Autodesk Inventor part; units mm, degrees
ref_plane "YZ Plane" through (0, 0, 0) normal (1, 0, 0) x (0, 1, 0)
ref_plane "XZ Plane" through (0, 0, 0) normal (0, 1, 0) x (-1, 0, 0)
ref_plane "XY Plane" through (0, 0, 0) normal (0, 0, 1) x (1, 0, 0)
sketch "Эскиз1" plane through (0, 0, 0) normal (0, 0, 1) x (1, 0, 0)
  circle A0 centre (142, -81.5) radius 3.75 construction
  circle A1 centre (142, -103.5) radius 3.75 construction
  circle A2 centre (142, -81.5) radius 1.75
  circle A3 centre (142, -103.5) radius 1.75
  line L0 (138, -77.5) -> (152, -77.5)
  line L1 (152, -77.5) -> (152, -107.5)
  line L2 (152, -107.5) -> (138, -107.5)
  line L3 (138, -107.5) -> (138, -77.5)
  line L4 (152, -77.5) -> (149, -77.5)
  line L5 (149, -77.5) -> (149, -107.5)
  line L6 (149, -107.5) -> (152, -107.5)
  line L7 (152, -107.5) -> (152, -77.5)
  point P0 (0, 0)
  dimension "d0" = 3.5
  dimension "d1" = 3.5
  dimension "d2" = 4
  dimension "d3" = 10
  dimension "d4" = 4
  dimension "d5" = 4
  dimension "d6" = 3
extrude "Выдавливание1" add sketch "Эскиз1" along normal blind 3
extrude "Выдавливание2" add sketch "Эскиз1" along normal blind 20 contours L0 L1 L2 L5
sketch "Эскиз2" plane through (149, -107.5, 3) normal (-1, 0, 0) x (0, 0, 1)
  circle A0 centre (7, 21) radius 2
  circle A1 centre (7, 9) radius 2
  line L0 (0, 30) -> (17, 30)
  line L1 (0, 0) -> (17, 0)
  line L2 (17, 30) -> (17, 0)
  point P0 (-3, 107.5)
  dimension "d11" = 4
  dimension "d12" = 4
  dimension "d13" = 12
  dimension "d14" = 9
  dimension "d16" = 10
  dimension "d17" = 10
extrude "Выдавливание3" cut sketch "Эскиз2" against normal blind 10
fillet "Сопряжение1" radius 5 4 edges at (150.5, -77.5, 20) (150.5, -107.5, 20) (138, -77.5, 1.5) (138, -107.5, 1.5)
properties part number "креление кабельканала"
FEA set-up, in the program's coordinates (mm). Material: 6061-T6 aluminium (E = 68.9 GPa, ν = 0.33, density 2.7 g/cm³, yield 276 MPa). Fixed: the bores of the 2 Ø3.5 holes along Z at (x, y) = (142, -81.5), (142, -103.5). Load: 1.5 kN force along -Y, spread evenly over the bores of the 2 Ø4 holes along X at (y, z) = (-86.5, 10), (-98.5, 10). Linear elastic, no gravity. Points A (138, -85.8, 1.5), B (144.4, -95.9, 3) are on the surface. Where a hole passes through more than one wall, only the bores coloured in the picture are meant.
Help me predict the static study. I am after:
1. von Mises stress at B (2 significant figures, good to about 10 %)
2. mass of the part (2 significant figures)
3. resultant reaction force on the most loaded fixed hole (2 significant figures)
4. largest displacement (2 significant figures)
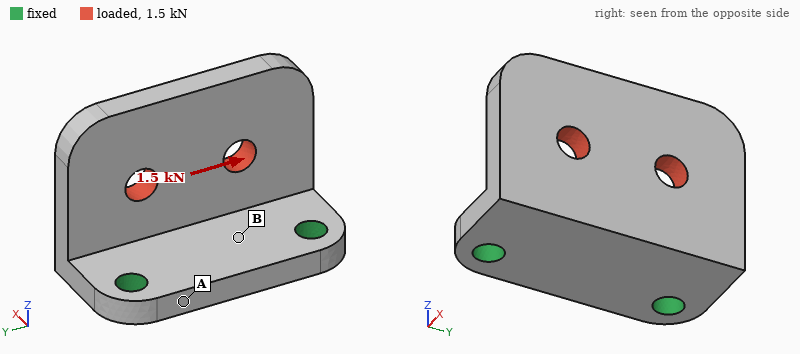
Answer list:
63 MPa
7.0 g
1.1 kN
85 µm
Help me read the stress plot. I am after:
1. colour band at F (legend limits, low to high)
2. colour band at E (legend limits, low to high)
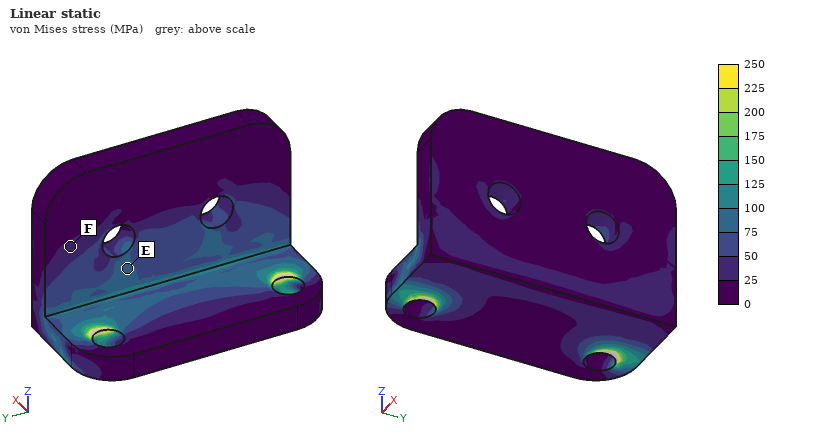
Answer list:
25 to 50 MPa
75 to 100 MPa
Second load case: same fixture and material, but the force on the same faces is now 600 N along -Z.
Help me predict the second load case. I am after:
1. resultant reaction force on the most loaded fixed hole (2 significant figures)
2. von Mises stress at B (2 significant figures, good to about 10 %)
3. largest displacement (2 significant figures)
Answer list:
300 N
34 MPa
94 µm
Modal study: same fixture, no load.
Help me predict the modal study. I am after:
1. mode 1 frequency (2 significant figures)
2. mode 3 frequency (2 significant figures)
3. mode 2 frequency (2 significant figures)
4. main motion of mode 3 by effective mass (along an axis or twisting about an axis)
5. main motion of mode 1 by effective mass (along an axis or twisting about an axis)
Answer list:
4400 Hz
14 kHz
9100 Hz
along Y
along X
